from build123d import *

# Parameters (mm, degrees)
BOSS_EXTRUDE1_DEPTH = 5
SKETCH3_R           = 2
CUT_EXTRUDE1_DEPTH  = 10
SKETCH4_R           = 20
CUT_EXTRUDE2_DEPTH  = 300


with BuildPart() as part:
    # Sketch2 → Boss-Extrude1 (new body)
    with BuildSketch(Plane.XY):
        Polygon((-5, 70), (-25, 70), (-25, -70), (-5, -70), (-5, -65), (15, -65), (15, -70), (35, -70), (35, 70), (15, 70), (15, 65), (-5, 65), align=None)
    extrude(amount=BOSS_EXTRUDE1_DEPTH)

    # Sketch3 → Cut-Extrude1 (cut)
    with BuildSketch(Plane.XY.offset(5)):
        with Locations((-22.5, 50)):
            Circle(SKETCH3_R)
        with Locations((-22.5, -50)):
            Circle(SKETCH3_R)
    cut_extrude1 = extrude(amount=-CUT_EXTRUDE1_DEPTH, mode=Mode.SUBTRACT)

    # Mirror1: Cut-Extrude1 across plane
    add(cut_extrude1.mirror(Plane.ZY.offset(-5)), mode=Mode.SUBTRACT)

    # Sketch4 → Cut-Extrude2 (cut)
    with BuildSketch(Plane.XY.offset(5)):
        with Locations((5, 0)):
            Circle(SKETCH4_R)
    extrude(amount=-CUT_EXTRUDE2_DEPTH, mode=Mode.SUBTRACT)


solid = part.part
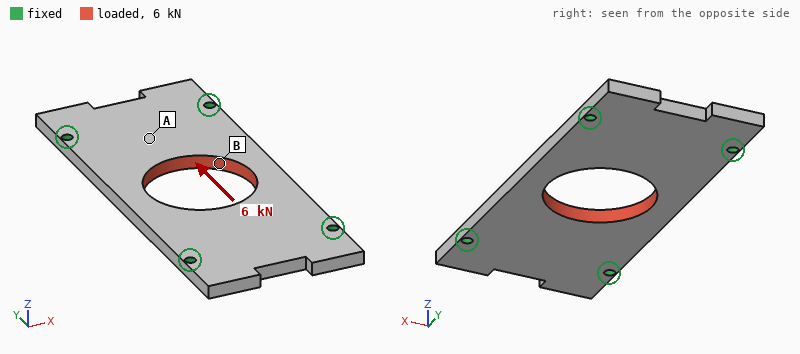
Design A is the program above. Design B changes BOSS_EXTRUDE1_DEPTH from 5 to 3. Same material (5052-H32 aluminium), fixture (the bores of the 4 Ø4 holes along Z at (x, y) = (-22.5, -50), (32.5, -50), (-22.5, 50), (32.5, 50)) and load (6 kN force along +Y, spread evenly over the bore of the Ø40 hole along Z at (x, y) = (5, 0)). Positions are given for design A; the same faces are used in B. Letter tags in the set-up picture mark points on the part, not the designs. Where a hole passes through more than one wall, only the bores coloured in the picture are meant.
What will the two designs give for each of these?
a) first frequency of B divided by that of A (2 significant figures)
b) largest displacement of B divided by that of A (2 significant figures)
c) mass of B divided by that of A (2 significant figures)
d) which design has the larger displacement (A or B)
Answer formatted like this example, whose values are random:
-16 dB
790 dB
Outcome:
0.62
1.7
0.60
B
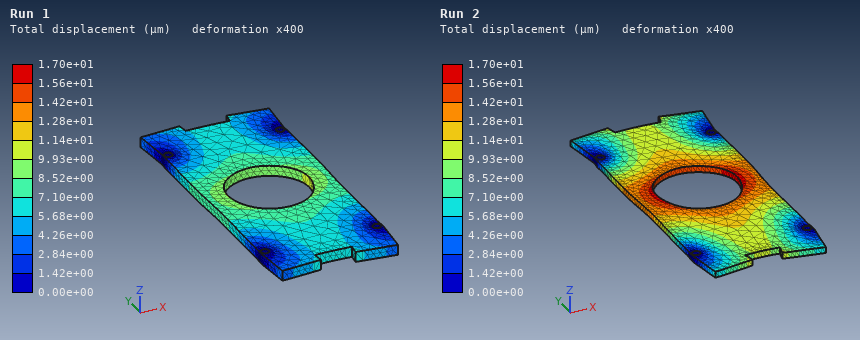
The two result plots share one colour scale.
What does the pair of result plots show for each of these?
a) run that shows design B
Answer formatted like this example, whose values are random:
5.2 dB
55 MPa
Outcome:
Run 2
